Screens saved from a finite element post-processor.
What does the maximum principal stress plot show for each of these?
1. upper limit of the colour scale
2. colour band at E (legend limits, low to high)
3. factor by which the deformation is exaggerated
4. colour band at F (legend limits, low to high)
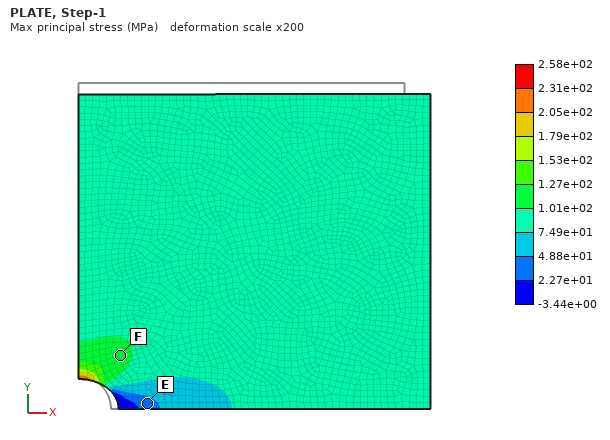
2.58e+02 MPa
2.27e+01 to 4.88e+01 MPa
200
1.01e+02 to 1.27e+02 MPa
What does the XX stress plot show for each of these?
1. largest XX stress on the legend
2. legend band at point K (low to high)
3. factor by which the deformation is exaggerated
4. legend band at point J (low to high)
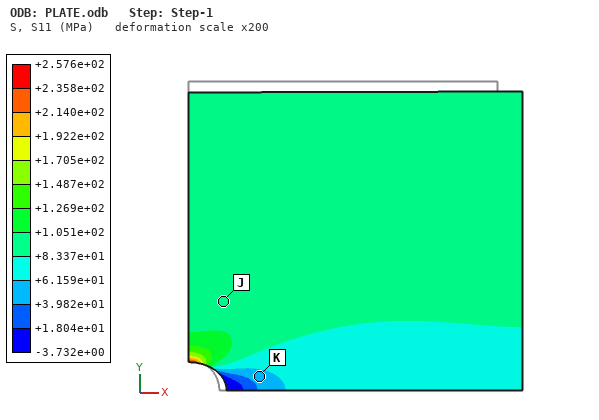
+2.576e+02 MPa
+3.982e+01 to +6.159e+01 MPa
200
+8.337e+01 to +1.051e+02 MPa
